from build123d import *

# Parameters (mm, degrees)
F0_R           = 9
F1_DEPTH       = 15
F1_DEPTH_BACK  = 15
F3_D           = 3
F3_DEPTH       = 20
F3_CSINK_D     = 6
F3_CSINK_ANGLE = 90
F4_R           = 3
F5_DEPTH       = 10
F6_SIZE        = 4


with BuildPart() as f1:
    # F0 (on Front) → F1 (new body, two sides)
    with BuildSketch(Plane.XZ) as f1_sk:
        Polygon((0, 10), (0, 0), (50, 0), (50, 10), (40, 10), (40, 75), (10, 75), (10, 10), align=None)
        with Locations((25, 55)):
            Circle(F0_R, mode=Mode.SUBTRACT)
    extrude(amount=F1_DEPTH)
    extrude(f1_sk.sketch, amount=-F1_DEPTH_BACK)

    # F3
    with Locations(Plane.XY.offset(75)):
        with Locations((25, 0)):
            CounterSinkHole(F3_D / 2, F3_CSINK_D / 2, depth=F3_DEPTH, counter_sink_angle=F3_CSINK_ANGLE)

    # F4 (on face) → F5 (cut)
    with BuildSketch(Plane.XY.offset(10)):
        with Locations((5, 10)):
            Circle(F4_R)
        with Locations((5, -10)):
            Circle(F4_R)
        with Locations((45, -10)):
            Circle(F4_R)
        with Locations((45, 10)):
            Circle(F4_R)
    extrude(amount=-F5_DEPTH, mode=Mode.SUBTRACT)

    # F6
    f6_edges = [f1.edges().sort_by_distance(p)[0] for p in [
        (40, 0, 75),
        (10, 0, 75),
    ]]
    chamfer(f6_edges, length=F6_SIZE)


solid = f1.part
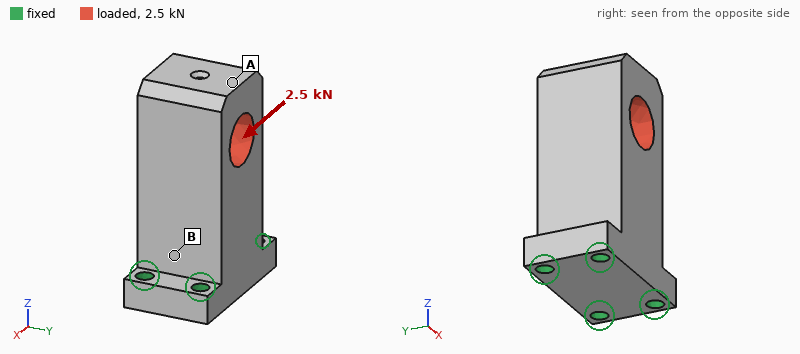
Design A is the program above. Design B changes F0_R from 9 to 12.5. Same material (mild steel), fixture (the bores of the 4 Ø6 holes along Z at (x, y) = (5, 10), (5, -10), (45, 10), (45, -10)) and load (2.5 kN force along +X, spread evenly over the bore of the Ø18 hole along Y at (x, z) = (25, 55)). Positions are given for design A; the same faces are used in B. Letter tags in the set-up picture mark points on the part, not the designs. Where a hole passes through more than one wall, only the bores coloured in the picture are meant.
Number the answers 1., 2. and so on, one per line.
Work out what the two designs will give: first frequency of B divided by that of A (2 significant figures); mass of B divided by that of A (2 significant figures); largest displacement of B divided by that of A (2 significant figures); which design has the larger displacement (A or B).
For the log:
1. 1.1
2. 0.89
3. 1.7
4. B
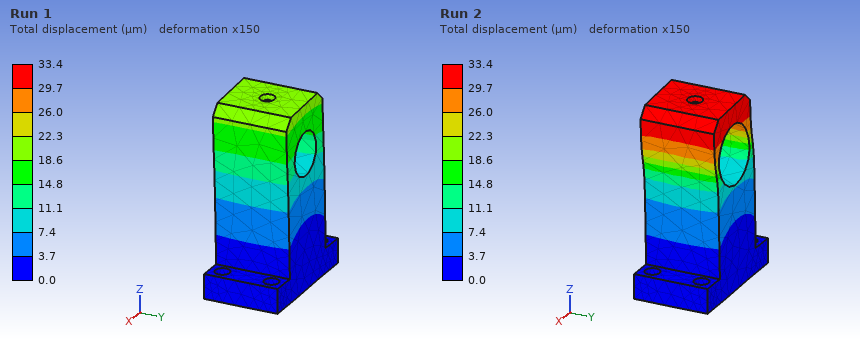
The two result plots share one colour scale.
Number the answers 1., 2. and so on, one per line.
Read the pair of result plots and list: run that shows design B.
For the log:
1. Run 2
